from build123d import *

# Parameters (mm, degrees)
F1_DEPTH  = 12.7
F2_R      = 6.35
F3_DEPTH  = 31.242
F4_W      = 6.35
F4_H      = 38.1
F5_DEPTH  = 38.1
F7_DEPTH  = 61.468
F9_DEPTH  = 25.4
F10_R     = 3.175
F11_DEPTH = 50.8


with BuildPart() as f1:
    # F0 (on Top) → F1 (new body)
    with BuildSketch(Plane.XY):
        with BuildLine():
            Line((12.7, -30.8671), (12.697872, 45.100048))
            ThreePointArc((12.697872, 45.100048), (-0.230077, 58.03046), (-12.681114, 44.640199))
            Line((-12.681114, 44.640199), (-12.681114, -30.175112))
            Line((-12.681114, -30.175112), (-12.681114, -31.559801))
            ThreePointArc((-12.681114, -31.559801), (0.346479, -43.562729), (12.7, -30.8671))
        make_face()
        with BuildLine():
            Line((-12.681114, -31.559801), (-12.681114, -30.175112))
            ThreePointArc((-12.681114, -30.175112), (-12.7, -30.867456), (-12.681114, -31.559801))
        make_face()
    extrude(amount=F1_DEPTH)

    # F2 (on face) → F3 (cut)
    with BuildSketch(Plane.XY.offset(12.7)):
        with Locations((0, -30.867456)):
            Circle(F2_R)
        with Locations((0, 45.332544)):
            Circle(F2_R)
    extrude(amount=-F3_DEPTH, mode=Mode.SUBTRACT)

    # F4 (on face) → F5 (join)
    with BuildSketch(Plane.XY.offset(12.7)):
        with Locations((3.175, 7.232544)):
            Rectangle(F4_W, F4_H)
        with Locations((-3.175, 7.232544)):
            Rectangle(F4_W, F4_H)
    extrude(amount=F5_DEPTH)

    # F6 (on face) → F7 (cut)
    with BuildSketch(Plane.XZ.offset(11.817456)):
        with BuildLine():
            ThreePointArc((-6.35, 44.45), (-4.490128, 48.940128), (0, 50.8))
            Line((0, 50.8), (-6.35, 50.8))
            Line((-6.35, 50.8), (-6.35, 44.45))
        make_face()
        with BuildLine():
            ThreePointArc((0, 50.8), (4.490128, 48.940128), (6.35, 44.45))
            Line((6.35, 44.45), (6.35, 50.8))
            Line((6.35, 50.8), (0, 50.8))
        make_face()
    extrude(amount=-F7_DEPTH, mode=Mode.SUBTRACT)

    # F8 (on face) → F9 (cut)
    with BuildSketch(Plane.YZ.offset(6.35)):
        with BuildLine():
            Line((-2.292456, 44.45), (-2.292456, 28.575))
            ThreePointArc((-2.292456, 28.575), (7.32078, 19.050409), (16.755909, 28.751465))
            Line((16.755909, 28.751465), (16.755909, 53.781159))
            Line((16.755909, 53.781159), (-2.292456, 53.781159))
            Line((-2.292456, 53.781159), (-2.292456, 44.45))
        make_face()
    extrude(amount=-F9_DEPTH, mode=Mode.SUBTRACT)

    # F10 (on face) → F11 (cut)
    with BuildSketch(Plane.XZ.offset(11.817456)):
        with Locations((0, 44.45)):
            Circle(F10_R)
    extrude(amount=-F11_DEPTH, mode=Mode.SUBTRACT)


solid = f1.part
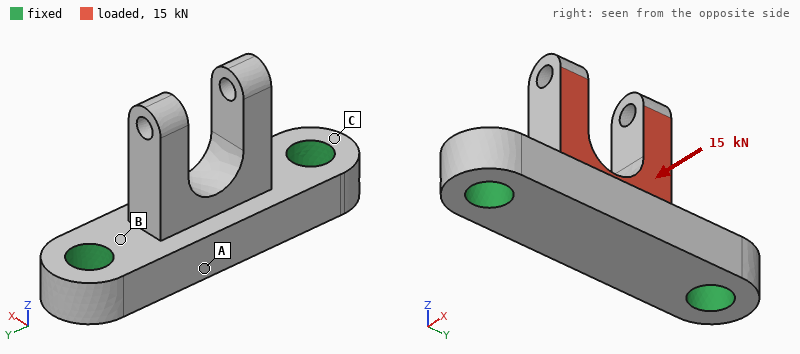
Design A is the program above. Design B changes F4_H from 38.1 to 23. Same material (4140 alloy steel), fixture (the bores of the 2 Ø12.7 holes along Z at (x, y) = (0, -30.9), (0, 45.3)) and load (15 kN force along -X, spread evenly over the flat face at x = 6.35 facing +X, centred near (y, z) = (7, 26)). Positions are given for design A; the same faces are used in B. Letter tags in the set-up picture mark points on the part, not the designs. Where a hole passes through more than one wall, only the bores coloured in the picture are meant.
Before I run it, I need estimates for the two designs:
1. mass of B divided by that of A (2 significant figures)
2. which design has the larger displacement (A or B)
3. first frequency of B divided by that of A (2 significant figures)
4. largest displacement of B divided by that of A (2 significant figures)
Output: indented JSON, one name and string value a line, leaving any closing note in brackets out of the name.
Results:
{
  "mass of B divided by that of A": "0.83",
  "which design has the larger displacement": "B",
  "first frequency of B divided by that of A": "0.54",
  "largest displacement of B divided by that of A": "1.4"
}
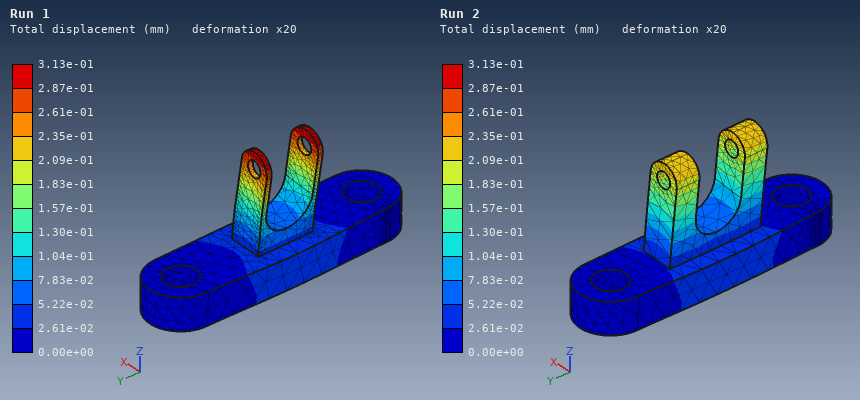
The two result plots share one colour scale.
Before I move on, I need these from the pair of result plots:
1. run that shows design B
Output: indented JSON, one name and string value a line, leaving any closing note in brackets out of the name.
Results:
{
  "run that shows design B": "Run 1"
}
